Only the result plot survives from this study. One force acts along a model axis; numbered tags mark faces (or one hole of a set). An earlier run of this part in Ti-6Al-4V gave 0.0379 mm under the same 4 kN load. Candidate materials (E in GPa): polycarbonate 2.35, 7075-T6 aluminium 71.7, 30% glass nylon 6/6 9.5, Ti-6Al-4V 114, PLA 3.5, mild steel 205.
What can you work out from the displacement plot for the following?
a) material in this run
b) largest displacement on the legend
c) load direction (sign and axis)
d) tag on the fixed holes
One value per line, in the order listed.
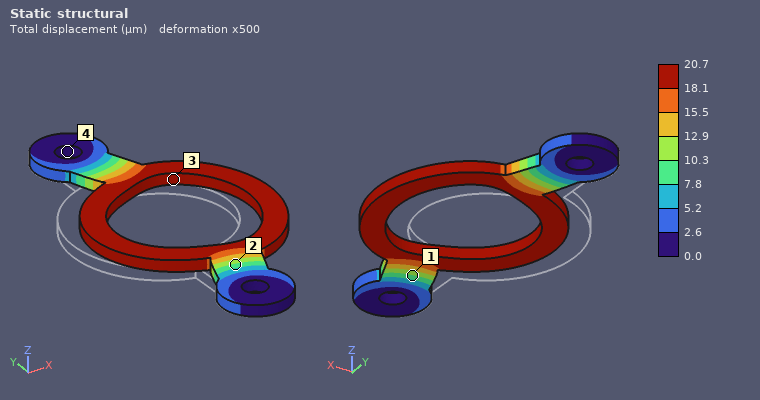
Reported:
mild steel
20.7 µm
+X
4
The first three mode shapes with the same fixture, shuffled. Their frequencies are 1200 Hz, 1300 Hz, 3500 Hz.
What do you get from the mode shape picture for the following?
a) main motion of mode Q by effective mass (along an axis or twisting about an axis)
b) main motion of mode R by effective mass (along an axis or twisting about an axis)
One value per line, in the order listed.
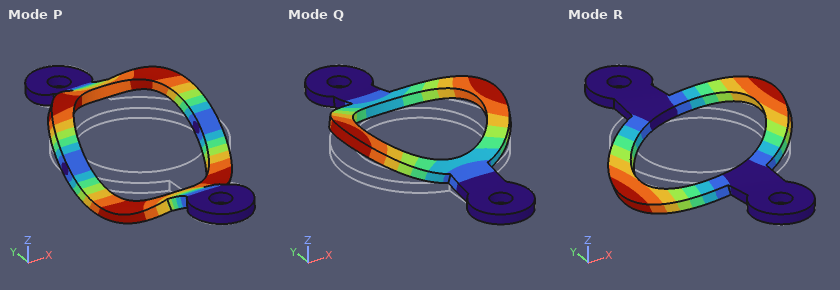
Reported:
along Z
twisting about Y
